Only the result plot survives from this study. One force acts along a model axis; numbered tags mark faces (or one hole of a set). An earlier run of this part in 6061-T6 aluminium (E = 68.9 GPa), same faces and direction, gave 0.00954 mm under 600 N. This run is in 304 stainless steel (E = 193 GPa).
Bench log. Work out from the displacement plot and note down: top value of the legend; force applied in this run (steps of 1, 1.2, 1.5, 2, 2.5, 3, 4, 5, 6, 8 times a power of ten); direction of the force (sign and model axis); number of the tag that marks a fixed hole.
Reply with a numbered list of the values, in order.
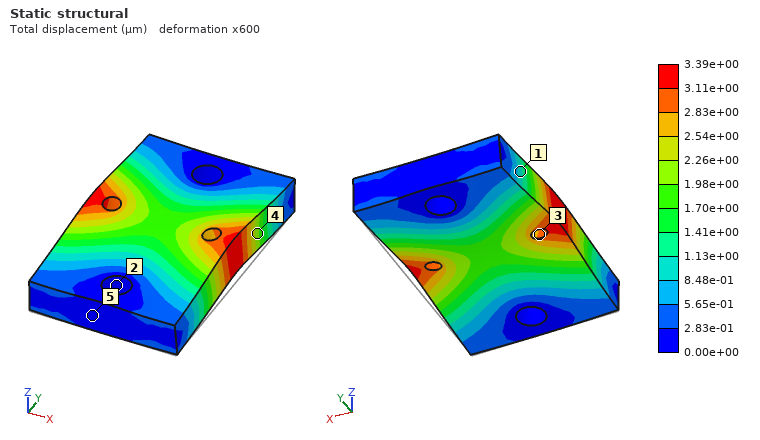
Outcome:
1. 3.39e+00 µm
2. 600 N
3. +Z
4. 2
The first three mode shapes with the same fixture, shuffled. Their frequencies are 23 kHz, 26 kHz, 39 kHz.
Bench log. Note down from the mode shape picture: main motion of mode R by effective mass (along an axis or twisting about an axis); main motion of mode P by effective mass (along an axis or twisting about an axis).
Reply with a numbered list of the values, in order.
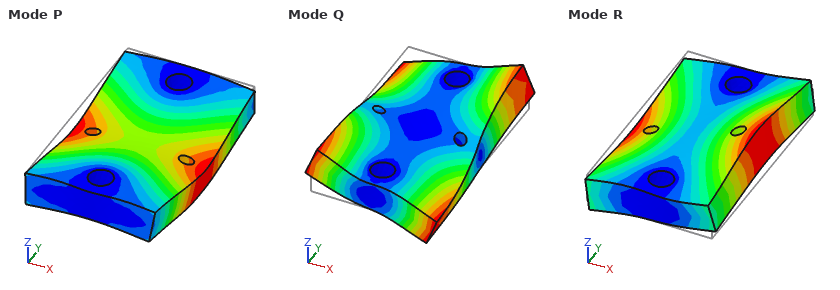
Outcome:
1. twisting about Y
2. along Z
